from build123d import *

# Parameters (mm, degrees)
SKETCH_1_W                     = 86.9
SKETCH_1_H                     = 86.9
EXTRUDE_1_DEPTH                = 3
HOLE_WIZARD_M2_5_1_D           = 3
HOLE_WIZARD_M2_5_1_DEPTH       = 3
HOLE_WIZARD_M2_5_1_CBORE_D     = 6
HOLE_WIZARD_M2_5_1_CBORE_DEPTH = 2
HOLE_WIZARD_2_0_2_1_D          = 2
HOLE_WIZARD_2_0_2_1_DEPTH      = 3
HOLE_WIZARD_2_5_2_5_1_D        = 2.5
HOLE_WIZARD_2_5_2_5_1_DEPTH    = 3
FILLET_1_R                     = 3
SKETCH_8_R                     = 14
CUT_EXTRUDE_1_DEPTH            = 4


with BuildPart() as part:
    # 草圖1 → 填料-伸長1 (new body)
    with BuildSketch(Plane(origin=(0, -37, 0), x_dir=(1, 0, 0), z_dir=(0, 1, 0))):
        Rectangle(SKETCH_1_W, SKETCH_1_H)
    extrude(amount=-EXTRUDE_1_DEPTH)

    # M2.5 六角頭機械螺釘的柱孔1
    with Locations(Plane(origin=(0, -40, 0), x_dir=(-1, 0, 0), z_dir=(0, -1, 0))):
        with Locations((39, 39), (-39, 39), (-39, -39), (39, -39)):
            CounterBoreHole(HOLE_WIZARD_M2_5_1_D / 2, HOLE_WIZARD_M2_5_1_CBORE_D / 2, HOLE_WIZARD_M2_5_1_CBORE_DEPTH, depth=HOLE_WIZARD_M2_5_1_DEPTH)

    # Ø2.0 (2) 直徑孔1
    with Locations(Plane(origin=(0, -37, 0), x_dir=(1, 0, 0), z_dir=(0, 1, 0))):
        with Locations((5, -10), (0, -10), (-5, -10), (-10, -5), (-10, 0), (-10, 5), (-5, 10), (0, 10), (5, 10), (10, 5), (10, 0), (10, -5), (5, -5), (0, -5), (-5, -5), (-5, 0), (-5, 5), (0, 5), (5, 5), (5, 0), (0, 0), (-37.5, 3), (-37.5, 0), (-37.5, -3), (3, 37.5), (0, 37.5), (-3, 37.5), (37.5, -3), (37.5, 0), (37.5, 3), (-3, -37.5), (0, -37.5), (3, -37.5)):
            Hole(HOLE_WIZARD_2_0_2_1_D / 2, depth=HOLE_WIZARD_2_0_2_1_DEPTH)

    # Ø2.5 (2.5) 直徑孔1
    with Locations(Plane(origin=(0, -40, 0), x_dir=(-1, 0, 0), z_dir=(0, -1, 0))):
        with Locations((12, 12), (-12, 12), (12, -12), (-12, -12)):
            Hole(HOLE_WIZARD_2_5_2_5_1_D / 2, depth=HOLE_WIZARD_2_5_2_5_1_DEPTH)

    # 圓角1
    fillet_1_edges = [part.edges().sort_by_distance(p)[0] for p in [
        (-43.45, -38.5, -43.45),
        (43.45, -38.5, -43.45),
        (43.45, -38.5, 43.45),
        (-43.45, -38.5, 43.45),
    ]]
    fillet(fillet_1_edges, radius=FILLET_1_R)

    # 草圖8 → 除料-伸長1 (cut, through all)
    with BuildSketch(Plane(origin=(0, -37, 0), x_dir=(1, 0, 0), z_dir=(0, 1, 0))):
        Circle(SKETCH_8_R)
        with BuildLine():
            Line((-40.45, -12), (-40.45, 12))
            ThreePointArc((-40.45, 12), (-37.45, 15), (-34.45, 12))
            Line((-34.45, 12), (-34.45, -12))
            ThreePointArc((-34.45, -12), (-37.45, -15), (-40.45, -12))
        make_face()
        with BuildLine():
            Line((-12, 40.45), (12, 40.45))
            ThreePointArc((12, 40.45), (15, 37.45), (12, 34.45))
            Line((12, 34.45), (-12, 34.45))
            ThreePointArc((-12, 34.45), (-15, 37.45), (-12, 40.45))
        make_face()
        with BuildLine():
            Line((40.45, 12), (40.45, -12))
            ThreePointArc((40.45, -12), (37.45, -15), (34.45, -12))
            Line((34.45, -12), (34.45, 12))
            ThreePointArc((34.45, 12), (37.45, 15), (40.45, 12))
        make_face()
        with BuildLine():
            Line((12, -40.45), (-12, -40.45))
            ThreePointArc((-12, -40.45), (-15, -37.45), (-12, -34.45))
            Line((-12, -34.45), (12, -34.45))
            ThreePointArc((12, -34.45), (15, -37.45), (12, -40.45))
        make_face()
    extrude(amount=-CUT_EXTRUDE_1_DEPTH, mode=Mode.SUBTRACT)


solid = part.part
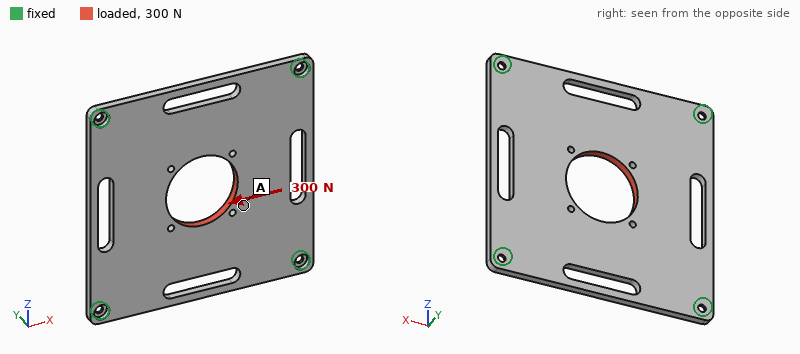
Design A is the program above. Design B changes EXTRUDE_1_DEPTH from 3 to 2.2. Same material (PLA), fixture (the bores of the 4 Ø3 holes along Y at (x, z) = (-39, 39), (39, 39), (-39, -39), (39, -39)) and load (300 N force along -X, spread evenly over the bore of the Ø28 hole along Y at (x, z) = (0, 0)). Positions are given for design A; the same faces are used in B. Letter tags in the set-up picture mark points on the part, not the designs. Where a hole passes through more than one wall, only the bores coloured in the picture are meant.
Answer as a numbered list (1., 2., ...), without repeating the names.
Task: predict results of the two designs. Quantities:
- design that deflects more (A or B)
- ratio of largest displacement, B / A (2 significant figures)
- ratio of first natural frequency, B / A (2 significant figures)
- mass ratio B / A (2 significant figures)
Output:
1. B
2. 1.2
3. 0.79
4. 0.73
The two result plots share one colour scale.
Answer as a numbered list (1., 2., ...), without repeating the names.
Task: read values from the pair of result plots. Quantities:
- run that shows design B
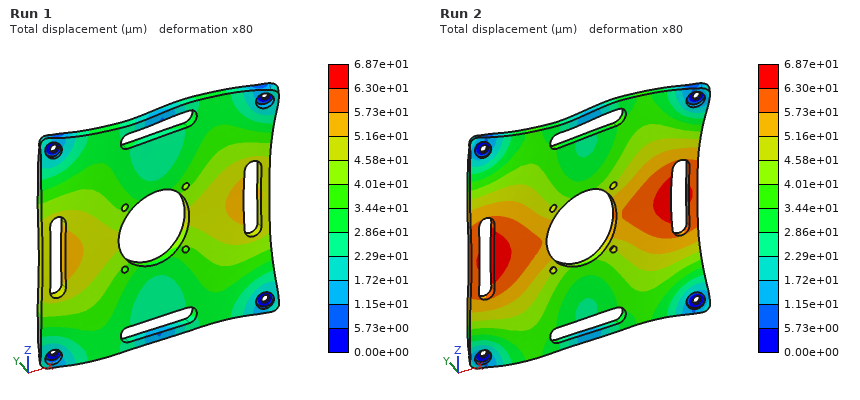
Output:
1. Run 2
